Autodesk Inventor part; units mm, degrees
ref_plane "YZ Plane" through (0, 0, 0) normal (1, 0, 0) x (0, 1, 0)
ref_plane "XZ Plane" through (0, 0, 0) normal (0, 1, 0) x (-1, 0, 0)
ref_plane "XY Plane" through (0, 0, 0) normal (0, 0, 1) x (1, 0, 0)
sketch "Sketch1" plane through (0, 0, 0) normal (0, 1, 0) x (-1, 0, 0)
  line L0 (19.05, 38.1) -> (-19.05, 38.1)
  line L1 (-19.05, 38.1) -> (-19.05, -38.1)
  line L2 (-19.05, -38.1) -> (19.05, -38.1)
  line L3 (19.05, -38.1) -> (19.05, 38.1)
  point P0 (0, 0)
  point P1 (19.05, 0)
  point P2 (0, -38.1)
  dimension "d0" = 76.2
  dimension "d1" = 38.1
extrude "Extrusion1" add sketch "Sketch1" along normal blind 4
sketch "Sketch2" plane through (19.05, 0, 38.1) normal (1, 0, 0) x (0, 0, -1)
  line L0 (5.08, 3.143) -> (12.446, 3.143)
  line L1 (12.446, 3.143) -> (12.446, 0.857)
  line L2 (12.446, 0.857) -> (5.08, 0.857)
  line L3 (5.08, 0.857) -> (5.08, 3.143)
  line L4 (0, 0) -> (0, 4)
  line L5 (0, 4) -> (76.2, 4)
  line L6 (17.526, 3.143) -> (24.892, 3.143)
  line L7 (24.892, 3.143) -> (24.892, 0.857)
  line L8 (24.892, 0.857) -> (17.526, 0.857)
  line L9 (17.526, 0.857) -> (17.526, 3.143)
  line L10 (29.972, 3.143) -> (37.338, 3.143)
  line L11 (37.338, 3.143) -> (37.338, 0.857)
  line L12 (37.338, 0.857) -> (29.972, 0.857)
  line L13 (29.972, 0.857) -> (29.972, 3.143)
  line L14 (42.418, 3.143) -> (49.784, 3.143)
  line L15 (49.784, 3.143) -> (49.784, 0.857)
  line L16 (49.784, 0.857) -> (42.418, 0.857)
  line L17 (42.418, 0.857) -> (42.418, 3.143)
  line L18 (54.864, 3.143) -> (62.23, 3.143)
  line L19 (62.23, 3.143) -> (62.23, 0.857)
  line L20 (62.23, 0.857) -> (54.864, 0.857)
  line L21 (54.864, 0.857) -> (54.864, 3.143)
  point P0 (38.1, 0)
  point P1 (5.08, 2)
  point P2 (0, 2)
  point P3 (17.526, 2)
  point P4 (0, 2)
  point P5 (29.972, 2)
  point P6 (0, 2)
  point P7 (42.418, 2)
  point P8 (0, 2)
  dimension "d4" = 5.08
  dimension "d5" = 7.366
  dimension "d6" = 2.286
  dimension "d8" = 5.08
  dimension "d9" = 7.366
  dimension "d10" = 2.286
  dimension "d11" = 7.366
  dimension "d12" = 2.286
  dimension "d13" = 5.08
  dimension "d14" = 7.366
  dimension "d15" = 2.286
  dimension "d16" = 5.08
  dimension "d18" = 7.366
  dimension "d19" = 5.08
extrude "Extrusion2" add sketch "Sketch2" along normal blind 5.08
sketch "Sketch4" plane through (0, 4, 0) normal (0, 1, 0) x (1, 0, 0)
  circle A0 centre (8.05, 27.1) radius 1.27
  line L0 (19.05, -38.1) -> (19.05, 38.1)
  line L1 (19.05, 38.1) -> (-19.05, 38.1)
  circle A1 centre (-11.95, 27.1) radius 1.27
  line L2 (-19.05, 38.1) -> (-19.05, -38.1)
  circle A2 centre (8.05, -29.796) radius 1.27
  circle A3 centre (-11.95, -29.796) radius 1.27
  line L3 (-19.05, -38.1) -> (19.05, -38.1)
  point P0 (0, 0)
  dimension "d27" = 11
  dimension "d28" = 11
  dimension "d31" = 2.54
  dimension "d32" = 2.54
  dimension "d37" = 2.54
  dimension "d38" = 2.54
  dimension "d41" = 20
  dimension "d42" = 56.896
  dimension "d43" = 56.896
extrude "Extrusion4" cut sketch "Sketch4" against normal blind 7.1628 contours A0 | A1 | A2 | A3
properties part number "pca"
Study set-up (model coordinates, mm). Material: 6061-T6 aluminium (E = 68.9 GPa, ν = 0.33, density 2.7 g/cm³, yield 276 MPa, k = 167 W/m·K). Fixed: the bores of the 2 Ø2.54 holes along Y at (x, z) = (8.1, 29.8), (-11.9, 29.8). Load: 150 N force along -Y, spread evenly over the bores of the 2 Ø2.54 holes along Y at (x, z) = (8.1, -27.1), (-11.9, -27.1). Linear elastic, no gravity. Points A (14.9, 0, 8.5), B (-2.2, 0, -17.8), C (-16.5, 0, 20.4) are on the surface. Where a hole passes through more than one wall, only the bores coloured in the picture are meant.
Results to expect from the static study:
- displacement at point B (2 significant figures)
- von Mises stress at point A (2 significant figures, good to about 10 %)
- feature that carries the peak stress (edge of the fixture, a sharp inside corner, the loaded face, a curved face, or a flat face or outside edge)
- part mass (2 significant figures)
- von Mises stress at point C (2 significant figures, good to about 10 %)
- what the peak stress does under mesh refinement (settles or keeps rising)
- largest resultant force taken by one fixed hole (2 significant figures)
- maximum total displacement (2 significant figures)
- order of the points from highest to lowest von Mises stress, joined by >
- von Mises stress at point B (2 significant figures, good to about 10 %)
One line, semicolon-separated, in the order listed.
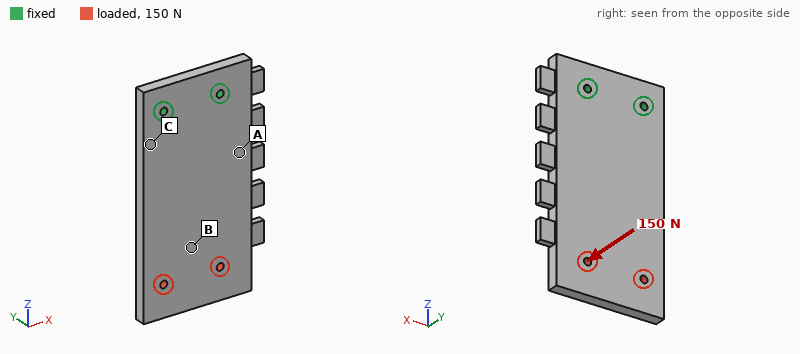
0.53 mm; 52 MPa; edge of the fixture; 32 g; 73 MPa; keeps rising; 78 N; 0.90 mm; C > A > B; 15 MPa
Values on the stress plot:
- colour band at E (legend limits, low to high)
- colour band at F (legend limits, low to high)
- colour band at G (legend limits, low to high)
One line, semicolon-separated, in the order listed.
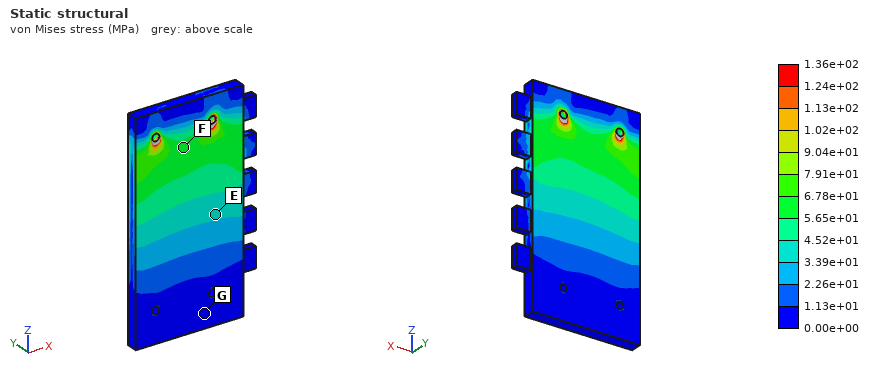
3.39e+01 to 4.52e+01 MPa; 5.65e+01 to 6.78e+01 MPa; 0.00e+00 to 1.13e+01 MPa
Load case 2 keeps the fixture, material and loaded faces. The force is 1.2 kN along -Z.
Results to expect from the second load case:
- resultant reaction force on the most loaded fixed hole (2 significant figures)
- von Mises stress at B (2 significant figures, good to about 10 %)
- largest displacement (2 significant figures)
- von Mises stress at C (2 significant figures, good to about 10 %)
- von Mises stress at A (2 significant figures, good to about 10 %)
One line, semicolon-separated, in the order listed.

600 N; 7.0 MPa; 9.6 µm; 9.5 MPa; 5.6 MPa
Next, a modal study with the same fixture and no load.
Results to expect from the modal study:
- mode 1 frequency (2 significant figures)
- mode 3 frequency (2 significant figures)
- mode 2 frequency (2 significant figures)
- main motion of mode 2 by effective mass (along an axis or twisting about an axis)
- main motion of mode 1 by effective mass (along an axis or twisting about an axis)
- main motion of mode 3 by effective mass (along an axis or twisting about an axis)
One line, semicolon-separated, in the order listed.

680 Hz; 4100 Hz; 2500 Hz; twisting about Z; along Y; along Y
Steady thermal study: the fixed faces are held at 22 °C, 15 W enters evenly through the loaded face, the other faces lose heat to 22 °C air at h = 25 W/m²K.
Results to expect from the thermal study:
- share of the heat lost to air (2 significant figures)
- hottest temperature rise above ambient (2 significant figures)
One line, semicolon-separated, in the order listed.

19 %; 33 K
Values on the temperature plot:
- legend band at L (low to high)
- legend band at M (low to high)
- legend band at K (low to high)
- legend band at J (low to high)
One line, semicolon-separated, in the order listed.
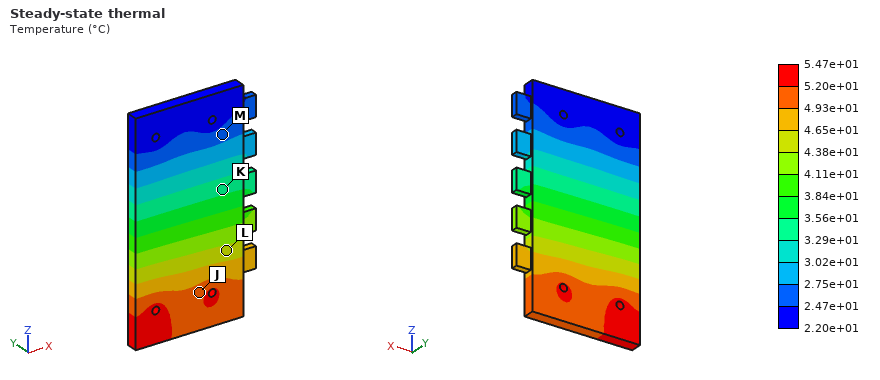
4.38e+01 to 4.65e+01 °C; 2.47e+01 to 2.75e+01 °C; 3.29e+01 to 3.56e+01 °C; 4.93e+01 to 5.20e+01 °C
